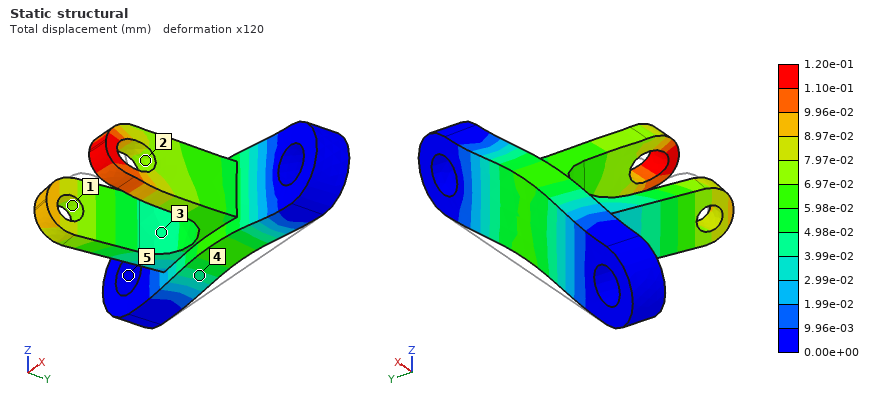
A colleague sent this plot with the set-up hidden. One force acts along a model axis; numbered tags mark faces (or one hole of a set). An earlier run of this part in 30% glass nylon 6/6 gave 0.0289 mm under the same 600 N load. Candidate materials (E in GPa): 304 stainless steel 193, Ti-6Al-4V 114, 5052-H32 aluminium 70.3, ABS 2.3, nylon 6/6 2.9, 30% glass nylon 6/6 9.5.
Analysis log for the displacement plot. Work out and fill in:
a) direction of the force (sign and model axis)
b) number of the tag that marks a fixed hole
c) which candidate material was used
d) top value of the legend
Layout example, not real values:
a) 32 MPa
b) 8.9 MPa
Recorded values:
a) -Y
b) 5
c) ABS
d) 1.20e-01 mm
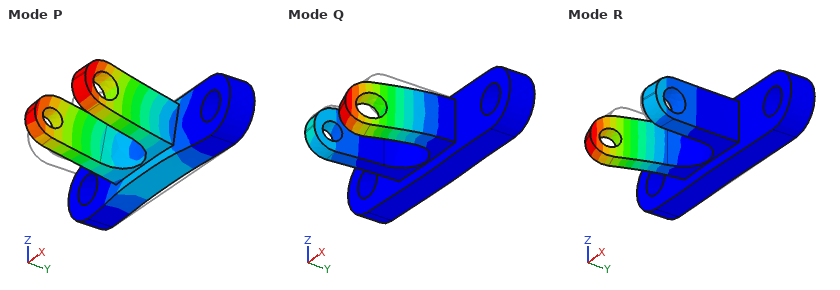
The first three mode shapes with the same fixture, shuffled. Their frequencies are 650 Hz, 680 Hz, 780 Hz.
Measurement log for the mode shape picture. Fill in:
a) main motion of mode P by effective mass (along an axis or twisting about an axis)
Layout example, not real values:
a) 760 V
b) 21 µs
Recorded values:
a) along Z
